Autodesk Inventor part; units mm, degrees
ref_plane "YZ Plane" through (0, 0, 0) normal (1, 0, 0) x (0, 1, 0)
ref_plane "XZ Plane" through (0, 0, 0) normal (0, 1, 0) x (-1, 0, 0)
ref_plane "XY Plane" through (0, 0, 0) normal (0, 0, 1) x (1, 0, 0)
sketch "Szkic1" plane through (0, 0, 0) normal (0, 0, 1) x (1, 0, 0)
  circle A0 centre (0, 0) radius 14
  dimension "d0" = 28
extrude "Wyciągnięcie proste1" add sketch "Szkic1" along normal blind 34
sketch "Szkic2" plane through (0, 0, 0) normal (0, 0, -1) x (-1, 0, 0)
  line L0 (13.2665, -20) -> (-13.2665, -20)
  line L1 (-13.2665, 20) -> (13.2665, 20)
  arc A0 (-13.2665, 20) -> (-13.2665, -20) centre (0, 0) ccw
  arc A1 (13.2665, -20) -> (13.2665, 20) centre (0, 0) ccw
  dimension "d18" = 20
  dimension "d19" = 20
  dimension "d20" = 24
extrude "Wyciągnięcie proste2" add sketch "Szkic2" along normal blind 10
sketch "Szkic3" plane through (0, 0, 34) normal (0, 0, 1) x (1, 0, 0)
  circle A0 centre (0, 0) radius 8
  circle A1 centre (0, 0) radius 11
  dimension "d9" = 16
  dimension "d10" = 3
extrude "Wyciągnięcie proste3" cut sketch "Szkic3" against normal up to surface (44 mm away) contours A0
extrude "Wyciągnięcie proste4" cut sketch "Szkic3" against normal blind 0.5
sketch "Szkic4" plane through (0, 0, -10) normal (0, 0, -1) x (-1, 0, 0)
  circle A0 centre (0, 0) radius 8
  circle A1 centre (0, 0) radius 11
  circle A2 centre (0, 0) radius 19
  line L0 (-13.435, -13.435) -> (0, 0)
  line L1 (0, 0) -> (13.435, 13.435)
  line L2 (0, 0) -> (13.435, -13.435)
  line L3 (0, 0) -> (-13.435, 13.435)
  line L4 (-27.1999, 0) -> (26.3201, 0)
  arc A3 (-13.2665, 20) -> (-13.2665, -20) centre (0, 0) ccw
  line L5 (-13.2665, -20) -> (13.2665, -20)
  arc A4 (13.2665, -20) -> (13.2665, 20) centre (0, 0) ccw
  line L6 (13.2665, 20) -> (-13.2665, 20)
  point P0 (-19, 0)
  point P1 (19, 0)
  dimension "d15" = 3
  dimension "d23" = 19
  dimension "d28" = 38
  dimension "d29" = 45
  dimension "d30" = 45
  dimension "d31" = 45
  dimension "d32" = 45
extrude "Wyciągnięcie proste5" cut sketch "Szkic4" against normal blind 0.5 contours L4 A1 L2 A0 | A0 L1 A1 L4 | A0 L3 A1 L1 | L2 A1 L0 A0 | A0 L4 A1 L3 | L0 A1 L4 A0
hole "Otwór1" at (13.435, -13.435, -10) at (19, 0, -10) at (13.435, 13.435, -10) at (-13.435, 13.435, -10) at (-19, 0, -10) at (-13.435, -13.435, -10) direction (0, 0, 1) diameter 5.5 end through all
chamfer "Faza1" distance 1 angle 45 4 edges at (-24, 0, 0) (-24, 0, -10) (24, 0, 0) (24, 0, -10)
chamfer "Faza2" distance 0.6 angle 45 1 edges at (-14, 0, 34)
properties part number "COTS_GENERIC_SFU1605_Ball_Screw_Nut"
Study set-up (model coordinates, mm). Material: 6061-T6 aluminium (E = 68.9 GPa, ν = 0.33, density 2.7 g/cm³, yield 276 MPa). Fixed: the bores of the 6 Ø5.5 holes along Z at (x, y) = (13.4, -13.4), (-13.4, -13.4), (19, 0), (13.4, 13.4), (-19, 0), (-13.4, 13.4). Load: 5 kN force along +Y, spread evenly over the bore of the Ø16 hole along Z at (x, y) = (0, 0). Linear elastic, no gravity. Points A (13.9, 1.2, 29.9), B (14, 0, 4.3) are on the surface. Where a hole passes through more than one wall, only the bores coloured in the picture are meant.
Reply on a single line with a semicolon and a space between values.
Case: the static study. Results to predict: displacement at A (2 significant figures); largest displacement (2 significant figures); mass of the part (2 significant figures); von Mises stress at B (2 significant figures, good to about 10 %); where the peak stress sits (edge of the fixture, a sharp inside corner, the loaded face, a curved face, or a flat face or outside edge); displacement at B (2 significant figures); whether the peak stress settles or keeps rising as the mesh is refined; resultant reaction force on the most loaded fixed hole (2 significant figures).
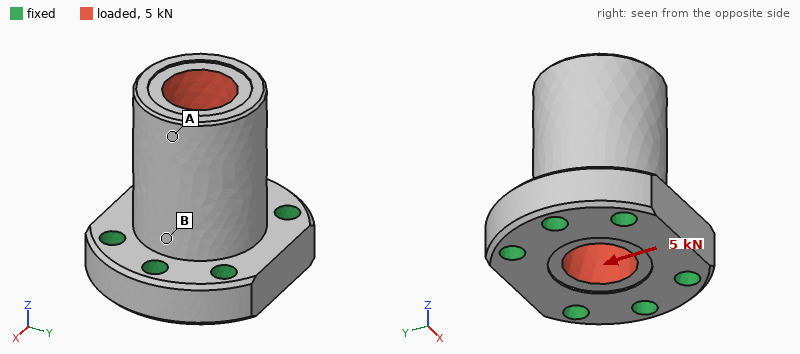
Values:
30 µm; 35 µm; 73 g; 17 MPa; edge of the fixture; 5.6 µm; keeps rising; 1.9 kN
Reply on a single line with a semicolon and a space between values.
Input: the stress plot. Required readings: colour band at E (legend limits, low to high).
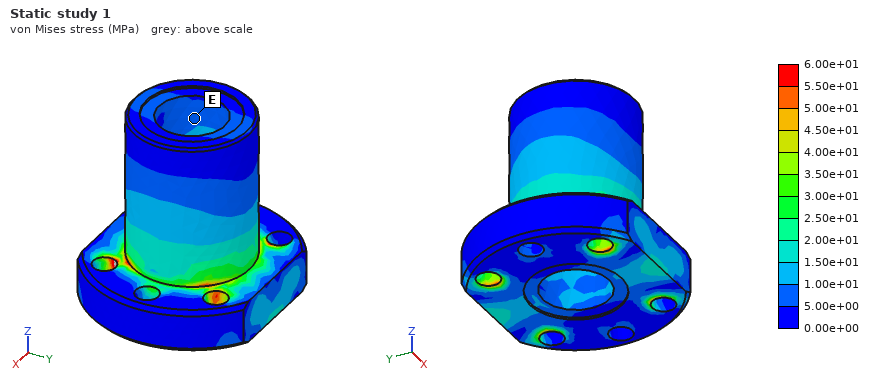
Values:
5.00e+00 to 1.00e+01 MPa
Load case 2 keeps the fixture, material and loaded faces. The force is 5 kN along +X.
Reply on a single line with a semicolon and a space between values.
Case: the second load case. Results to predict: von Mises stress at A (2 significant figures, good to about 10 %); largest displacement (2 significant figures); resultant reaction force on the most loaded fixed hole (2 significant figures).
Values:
4.0 MPa; 30 µm; 1.6 kN
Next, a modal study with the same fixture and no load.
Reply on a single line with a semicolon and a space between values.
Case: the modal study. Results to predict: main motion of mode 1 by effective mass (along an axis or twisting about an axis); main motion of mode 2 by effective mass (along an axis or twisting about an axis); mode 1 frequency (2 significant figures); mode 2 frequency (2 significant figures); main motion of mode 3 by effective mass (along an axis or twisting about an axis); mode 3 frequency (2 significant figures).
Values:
along Y; along X; 10 kHz; 11 kHz; twisting about Z; 21 kHz
